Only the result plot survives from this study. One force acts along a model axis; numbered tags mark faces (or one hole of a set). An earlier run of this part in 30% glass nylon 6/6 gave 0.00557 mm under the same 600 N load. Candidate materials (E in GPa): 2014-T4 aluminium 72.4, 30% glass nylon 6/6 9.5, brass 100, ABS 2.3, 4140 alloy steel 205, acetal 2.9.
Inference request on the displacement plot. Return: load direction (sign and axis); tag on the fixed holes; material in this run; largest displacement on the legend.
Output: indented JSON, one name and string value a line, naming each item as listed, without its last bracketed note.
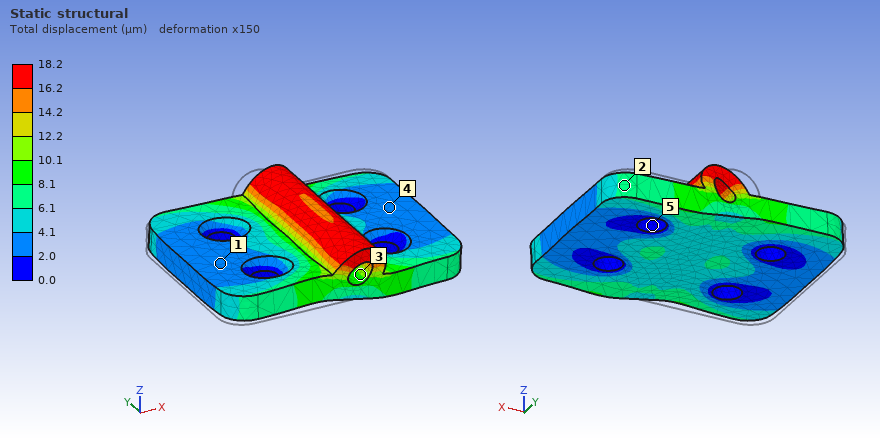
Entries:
{
  "load direction": "+X",
  "tag on the fixed holes": "5",
  "material in this run": "acetal",
  "largest displacement on the legend": "18.2 µm"
}
